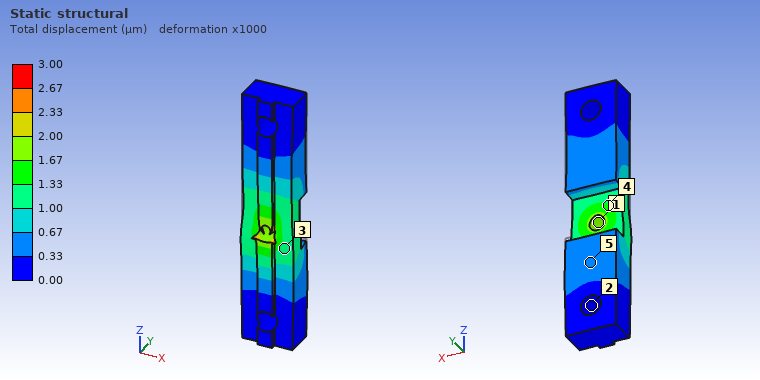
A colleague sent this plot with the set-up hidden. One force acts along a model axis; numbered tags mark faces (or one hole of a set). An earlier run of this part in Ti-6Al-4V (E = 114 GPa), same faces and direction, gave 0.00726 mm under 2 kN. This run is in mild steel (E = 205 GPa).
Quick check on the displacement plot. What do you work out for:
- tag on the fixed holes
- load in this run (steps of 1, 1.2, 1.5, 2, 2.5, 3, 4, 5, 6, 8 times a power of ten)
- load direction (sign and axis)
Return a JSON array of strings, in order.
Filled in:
["2", "1.5 kN", "-Z"]
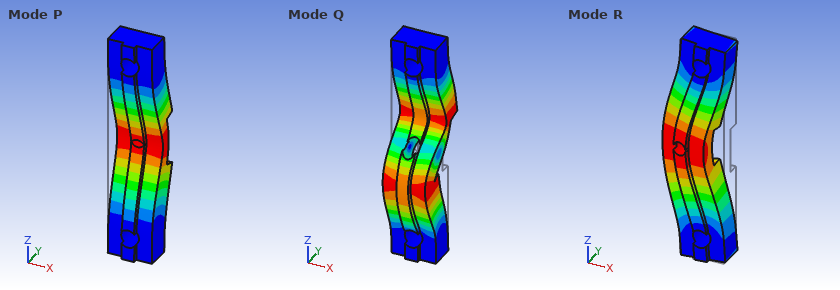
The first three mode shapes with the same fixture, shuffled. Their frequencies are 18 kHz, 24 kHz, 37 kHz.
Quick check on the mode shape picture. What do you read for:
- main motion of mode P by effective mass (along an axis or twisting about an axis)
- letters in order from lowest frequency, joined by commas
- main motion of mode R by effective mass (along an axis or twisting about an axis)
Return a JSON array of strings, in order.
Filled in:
["along Y", "P, R, Q", "along X"]
